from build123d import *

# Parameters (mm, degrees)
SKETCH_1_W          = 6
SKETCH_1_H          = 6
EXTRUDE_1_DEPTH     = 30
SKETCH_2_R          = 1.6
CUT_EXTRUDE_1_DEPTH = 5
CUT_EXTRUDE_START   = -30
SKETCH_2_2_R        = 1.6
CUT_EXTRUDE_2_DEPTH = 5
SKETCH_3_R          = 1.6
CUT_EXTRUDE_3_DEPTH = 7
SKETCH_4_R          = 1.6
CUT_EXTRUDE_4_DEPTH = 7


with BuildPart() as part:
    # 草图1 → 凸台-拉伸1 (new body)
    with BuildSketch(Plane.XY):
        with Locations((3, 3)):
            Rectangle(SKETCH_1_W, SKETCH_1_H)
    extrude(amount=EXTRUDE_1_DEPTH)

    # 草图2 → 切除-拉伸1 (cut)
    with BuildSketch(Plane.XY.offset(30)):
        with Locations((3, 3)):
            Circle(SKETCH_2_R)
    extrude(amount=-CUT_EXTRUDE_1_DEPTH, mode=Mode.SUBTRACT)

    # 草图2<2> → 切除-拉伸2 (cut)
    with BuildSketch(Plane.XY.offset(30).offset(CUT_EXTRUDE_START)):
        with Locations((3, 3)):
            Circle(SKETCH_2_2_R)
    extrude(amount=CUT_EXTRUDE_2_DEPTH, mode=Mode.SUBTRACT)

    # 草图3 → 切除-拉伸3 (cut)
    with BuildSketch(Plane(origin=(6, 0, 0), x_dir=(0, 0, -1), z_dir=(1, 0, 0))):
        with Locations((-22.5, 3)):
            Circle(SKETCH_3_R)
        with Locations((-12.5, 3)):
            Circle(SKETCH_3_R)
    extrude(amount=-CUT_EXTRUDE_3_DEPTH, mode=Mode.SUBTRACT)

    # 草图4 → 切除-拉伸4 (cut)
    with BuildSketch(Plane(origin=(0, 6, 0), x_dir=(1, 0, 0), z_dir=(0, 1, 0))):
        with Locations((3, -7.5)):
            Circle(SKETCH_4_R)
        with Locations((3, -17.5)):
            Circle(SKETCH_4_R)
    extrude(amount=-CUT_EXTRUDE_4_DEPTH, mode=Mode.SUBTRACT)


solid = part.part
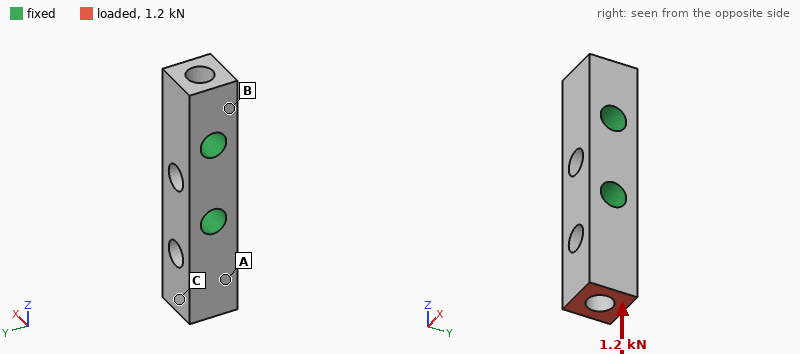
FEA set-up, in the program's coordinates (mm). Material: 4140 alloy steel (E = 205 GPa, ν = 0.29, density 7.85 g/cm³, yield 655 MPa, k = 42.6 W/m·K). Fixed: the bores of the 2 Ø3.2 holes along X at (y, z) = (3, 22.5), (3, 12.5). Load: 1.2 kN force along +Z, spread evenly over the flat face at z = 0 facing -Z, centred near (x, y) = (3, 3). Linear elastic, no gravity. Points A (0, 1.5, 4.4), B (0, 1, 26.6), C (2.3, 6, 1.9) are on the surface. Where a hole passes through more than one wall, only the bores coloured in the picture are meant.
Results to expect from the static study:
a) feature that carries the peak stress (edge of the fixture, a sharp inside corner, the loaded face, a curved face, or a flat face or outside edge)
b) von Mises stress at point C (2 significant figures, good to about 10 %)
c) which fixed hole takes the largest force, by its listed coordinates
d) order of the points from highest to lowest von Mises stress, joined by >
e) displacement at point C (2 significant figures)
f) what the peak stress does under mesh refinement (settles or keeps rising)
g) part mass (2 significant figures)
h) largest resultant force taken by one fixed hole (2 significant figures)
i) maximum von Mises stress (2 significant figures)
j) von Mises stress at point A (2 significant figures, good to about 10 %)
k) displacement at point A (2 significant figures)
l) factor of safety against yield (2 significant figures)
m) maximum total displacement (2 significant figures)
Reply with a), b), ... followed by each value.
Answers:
a) a curved face
b) 38 MPa
c) (3, 12.5)
d) A > C > B
e) 2.6 µm
f) settles
g) 6.3 g
h) 1.2 kN
i) 140 MPa
j) 58 MPa
k) 2.0 µm
l) 4.6
m) 3.0 µm
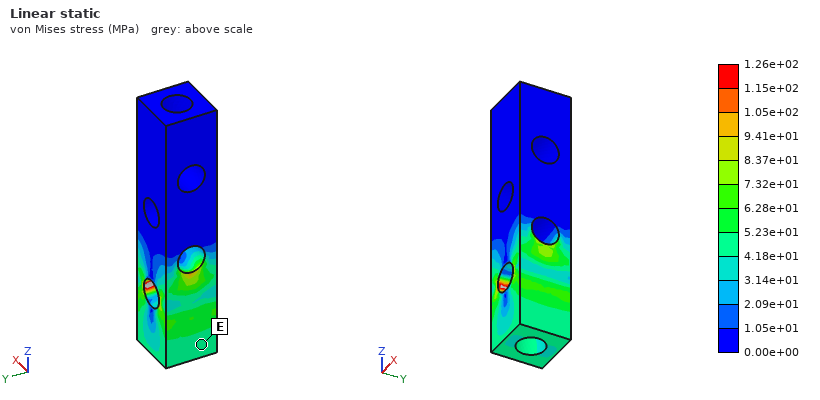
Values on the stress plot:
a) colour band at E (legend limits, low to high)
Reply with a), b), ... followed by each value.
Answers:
a) 4.18e+01 to 5.23e+01 MPa
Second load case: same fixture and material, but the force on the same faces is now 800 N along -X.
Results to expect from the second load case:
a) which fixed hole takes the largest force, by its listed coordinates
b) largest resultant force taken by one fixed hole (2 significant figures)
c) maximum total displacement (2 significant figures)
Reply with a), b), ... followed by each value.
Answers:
a) (3, 12.5)
b) 820 N
c) 32 µm
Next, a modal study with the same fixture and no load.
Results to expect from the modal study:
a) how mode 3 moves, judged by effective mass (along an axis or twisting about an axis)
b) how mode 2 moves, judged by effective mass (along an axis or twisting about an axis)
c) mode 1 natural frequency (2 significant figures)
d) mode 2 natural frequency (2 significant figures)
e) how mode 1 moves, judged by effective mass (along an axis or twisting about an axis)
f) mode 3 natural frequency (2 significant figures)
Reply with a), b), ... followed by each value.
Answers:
a) twisting about Z
b) along X
c) 26 kHz
d) 29 kHz
e) along Y
f) 53 kHz
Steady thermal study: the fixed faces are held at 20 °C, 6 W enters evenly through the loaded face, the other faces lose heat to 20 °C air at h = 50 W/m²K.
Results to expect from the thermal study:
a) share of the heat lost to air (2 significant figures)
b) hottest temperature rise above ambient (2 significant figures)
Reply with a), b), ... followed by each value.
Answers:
a) 9.9 %
b) 60 K
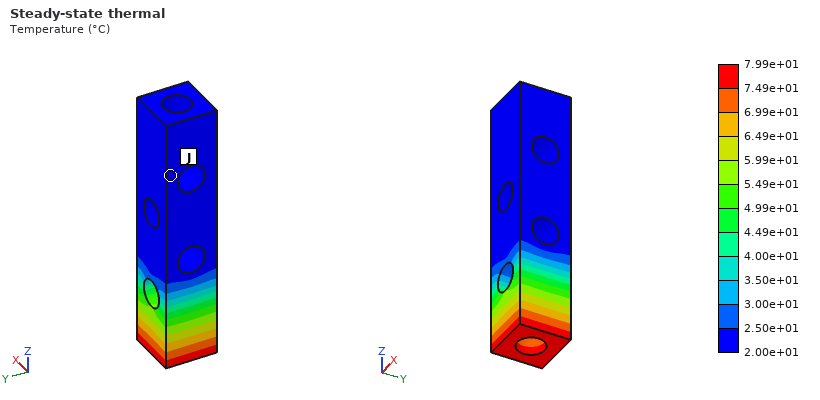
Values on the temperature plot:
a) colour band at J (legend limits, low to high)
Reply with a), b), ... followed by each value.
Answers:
a) 2.00e+01 to 2.50e+01 °C
